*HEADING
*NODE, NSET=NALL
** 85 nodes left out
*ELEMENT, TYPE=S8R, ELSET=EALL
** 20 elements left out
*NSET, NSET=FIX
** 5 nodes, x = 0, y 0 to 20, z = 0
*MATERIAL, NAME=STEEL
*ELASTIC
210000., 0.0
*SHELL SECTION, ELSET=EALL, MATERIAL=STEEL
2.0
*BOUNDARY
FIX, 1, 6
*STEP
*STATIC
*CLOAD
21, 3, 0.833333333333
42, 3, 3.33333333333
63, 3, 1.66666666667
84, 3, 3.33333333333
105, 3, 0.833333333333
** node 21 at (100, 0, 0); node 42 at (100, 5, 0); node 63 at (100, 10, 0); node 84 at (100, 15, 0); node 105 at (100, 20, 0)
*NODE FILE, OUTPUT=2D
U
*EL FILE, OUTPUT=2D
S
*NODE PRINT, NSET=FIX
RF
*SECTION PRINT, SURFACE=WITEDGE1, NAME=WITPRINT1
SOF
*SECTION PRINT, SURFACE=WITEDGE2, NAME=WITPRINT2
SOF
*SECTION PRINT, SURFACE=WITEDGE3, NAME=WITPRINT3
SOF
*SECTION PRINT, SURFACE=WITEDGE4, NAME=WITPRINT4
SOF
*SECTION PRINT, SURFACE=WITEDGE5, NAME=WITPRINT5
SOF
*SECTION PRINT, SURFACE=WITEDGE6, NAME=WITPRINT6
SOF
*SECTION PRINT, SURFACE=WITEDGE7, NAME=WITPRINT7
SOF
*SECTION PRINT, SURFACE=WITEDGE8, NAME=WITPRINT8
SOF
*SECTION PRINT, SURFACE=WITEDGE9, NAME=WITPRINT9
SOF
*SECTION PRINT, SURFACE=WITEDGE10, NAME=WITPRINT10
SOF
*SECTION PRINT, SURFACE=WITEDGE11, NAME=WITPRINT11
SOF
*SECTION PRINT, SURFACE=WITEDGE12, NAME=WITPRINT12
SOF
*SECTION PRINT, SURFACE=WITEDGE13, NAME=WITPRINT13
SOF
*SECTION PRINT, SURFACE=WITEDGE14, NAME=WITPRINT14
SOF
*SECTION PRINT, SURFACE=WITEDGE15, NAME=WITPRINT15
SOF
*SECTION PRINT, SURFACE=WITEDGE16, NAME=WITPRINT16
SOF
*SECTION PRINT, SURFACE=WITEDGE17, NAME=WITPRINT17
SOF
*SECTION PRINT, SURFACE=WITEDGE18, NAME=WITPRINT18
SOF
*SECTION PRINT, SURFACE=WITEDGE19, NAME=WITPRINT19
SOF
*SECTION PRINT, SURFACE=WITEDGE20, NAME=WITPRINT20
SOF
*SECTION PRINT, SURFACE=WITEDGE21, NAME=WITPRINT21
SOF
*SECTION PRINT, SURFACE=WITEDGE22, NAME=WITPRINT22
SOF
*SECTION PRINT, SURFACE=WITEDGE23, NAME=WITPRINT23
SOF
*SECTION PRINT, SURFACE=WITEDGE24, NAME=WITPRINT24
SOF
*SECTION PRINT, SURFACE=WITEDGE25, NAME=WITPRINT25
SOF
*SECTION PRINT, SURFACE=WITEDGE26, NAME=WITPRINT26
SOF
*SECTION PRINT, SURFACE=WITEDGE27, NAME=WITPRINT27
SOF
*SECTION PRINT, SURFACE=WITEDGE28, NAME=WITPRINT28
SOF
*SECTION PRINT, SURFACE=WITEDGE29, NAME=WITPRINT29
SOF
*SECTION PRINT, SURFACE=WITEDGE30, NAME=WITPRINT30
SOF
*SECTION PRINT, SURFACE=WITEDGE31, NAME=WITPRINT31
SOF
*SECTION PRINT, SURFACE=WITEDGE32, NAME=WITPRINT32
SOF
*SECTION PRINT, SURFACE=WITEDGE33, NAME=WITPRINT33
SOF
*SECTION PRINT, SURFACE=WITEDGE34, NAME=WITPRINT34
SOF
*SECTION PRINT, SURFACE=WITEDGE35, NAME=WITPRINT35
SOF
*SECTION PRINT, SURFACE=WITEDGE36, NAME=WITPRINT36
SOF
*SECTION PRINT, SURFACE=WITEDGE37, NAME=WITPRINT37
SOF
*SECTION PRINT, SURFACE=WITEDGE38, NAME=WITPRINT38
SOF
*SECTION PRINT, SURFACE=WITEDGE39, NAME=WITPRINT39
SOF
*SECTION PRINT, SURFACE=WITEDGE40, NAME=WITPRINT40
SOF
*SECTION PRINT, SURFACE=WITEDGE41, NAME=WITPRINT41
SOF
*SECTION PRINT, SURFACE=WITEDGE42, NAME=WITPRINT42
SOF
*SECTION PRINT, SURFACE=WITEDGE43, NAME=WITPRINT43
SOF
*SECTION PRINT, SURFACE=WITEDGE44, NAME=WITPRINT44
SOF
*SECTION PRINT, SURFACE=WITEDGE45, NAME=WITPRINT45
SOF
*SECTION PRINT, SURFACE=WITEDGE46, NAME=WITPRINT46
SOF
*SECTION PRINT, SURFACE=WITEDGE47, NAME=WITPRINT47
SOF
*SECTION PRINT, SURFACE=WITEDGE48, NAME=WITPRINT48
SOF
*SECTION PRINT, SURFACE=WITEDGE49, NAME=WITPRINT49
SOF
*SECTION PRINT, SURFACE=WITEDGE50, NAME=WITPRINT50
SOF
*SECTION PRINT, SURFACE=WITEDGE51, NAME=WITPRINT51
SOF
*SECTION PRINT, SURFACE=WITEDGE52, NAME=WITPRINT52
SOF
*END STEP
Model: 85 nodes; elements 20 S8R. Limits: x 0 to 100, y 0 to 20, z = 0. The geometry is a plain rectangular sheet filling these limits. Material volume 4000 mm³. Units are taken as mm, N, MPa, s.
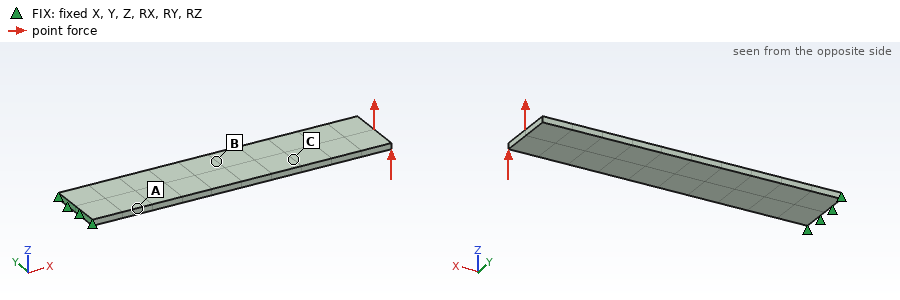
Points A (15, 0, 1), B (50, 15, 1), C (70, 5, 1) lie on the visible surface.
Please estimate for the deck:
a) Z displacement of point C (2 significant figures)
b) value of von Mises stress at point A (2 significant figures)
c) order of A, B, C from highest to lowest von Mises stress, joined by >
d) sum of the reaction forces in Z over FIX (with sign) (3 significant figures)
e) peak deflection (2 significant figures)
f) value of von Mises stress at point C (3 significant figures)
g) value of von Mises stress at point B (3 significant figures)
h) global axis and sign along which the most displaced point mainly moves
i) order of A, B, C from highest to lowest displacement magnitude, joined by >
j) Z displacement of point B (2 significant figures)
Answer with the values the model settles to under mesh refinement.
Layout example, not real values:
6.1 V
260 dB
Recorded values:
0.67 mm
64 MPa
A > B > C
-10.0 N
1.2 mm
22.5 MPa
37.5 MPa
+Z
C > B > A
0.37 mm
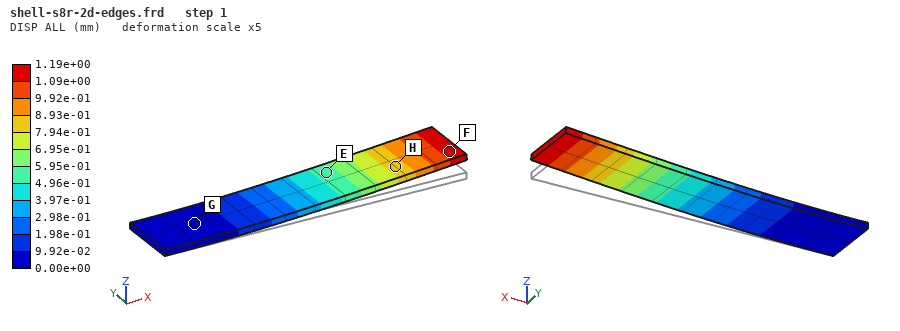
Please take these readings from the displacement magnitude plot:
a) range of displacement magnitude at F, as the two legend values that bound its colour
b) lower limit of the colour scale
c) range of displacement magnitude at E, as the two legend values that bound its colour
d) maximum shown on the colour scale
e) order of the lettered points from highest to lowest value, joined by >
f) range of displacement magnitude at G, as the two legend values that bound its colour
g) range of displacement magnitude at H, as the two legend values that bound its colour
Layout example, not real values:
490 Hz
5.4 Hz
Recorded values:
1.09e+00 to 1.19e+00 mm
0.00e+00 mm
4.96e-01 to 5.95e-01 mm
1.19e+00 mm
F > H > E > G
0.00e+00 to 9.92e-02 mm
7.94e-01 to 8.93e-01 mm
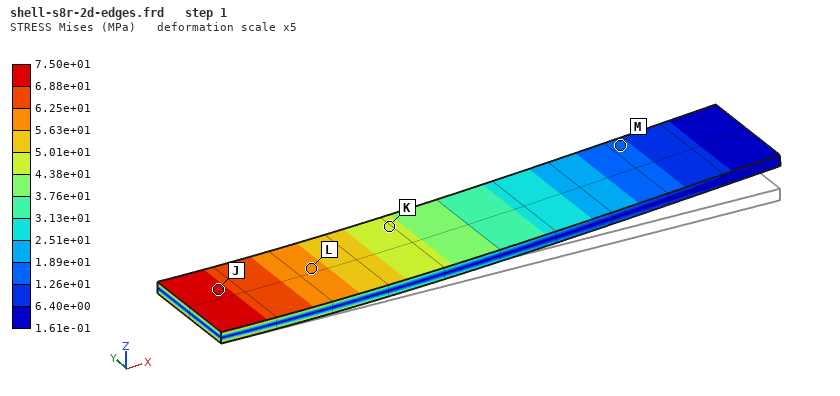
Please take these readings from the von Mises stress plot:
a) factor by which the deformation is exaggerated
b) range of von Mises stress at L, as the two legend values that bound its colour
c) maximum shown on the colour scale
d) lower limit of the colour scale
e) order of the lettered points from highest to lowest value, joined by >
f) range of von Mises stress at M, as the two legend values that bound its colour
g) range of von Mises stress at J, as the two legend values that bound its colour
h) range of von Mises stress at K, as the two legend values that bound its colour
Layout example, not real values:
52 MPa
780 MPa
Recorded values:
5
5.63e+01 to 6.25e+01 MPa
7.50e+01 MPa
1.61e-01 MPa
J > L > K > M
1.26e+01 to 1.89e+01 MPa
6.88e+01 to 7.50e+01 MPa
4.38e+01 to 5.01e+01 MPa
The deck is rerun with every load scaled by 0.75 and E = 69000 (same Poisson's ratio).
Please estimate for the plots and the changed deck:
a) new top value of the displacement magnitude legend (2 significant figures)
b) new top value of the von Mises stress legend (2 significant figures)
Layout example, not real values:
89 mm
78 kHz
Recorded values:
2.7 mm
56 MPa
